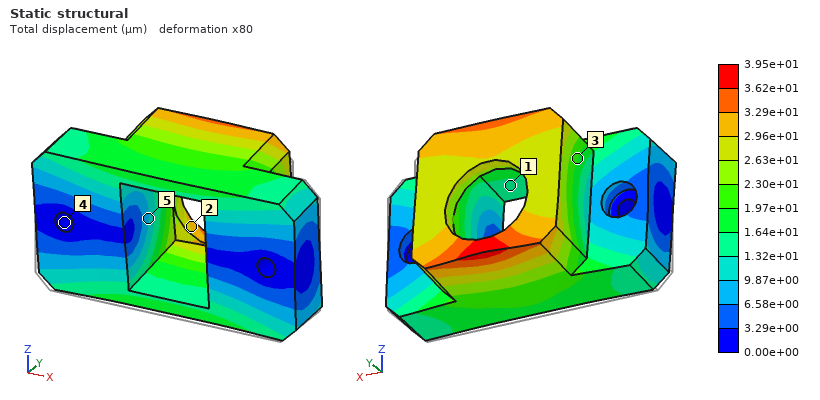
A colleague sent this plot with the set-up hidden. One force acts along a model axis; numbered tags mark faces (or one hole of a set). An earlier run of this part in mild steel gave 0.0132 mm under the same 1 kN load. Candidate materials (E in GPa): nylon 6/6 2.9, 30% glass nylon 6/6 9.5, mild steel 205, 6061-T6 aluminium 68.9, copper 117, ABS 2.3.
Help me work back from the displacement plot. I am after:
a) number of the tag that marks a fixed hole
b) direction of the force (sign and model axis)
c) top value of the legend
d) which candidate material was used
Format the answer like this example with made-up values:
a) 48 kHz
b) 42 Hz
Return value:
a) 4
b) +Z
c) 3.95e+01 µm
d) 6061-T6 aluminium
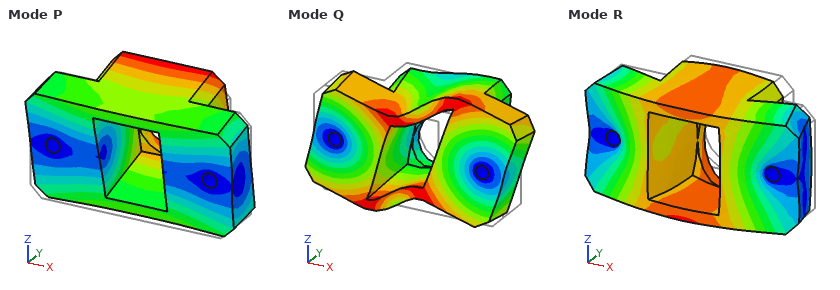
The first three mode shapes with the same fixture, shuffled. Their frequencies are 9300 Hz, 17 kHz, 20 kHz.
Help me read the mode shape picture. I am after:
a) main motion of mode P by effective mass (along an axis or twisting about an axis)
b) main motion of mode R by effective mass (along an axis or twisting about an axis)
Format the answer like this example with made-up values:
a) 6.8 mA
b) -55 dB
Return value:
a) along Z
b) along Y
